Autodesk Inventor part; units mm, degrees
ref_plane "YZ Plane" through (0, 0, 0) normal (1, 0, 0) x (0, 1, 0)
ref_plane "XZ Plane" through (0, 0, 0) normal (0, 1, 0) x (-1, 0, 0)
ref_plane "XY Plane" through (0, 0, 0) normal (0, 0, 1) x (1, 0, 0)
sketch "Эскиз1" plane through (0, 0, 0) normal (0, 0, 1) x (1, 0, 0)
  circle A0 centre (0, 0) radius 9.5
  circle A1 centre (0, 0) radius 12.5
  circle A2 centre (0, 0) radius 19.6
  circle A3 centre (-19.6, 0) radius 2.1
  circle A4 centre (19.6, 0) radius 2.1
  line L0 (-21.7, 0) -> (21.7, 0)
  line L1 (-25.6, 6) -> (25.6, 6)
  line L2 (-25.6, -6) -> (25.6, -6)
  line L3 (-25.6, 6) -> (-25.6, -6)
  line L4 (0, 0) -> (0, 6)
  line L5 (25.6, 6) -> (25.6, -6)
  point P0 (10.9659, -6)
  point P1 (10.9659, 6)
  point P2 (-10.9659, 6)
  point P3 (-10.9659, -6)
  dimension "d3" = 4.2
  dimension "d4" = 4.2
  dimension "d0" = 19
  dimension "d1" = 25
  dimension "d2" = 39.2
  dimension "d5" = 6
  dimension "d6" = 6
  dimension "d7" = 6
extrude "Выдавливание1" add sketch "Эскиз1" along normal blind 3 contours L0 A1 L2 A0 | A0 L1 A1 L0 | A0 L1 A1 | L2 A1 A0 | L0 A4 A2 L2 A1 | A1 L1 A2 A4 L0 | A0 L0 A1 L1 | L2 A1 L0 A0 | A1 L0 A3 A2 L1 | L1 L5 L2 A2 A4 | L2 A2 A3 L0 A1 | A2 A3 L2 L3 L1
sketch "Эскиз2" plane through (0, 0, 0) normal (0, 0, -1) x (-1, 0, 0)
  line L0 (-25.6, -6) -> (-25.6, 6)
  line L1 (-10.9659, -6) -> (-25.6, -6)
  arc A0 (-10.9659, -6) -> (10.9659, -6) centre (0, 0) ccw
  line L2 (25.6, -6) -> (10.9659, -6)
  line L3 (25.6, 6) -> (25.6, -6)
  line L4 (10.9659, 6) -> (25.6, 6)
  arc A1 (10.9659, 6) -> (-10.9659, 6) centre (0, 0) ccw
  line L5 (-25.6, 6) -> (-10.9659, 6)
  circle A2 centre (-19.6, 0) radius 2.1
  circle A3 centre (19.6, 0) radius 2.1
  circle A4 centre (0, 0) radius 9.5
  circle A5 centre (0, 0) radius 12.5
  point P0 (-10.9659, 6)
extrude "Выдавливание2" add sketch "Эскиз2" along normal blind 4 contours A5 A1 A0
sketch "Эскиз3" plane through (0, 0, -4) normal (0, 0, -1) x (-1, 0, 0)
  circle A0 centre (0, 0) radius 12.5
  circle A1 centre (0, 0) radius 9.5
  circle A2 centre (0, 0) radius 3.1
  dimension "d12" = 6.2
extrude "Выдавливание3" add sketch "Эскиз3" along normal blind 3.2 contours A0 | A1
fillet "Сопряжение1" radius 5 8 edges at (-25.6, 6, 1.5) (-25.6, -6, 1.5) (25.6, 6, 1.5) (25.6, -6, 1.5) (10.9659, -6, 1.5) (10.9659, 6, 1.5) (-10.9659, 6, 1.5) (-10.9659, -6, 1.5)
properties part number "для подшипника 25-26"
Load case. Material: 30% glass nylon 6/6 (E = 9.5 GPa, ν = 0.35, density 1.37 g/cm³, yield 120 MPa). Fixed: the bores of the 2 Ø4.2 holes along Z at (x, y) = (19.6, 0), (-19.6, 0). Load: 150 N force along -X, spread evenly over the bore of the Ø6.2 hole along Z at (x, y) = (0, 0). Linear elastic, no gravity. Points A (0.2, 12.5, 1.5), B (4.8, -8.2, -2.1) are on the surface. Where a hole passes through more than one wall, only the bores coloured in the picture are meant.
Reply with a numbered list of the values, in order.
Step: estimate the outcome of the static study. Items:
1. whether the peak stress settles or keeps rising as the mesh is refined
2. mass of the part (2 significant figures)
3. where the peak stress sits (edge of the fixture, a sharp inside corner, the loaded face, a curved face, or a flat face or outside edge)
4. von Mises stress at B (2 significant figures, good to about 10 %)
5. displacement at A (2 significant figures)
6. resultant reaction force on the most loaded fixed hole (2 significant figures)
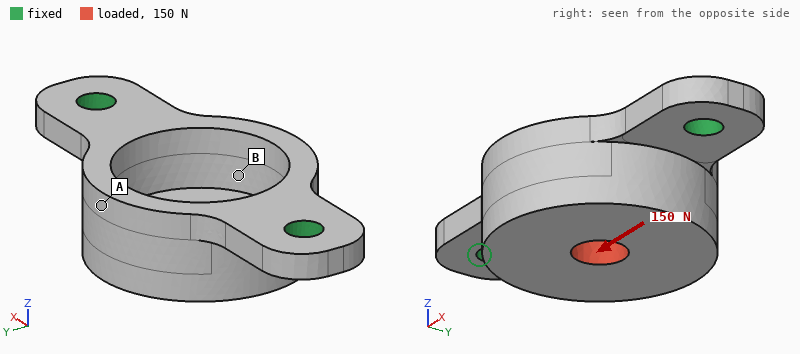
1. keeps rising
2. 5.2 g
3. edge of the fixture
4. 2.3 MPa
5. 4.0 µm
6. 83 N
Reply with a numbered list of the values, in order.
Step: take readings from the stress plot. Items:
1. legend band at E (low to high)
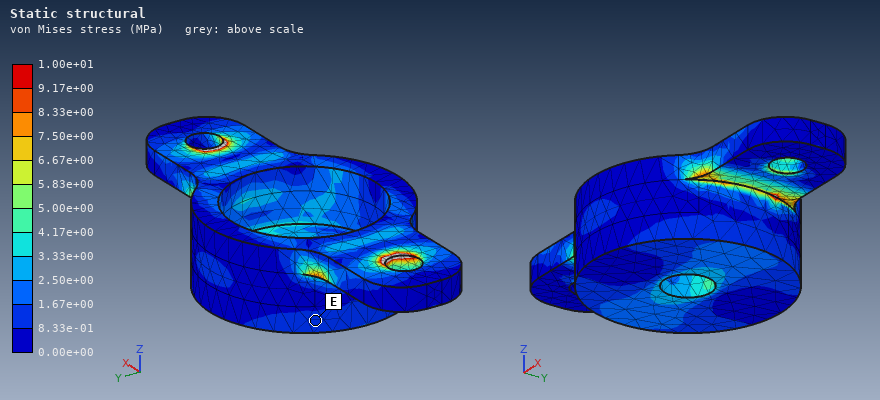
1. 8.33e-01 to 1.67e+00 MPa
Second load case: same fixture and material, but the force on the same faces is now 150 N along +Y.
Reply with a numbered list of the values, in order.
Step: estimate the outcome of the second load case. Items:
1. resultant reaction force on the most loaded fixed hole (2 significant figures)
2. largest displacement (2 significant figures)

1. 75 N
2. 0.15 mm
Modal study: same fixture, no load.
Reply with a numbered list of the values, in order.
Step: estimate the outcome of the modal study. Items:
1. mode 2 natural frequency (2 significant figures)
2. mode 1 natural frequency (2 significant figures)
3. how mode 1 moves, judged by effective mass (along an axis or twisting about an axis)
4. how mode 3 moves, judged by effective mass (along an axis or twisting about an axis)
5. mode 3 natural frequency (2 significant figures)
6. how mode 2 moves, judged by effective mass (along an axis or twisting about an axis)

1. 6300 Hz
2. 2900 Hz
3. along Y
4. along X
5. 11 kHz
6. along Z
